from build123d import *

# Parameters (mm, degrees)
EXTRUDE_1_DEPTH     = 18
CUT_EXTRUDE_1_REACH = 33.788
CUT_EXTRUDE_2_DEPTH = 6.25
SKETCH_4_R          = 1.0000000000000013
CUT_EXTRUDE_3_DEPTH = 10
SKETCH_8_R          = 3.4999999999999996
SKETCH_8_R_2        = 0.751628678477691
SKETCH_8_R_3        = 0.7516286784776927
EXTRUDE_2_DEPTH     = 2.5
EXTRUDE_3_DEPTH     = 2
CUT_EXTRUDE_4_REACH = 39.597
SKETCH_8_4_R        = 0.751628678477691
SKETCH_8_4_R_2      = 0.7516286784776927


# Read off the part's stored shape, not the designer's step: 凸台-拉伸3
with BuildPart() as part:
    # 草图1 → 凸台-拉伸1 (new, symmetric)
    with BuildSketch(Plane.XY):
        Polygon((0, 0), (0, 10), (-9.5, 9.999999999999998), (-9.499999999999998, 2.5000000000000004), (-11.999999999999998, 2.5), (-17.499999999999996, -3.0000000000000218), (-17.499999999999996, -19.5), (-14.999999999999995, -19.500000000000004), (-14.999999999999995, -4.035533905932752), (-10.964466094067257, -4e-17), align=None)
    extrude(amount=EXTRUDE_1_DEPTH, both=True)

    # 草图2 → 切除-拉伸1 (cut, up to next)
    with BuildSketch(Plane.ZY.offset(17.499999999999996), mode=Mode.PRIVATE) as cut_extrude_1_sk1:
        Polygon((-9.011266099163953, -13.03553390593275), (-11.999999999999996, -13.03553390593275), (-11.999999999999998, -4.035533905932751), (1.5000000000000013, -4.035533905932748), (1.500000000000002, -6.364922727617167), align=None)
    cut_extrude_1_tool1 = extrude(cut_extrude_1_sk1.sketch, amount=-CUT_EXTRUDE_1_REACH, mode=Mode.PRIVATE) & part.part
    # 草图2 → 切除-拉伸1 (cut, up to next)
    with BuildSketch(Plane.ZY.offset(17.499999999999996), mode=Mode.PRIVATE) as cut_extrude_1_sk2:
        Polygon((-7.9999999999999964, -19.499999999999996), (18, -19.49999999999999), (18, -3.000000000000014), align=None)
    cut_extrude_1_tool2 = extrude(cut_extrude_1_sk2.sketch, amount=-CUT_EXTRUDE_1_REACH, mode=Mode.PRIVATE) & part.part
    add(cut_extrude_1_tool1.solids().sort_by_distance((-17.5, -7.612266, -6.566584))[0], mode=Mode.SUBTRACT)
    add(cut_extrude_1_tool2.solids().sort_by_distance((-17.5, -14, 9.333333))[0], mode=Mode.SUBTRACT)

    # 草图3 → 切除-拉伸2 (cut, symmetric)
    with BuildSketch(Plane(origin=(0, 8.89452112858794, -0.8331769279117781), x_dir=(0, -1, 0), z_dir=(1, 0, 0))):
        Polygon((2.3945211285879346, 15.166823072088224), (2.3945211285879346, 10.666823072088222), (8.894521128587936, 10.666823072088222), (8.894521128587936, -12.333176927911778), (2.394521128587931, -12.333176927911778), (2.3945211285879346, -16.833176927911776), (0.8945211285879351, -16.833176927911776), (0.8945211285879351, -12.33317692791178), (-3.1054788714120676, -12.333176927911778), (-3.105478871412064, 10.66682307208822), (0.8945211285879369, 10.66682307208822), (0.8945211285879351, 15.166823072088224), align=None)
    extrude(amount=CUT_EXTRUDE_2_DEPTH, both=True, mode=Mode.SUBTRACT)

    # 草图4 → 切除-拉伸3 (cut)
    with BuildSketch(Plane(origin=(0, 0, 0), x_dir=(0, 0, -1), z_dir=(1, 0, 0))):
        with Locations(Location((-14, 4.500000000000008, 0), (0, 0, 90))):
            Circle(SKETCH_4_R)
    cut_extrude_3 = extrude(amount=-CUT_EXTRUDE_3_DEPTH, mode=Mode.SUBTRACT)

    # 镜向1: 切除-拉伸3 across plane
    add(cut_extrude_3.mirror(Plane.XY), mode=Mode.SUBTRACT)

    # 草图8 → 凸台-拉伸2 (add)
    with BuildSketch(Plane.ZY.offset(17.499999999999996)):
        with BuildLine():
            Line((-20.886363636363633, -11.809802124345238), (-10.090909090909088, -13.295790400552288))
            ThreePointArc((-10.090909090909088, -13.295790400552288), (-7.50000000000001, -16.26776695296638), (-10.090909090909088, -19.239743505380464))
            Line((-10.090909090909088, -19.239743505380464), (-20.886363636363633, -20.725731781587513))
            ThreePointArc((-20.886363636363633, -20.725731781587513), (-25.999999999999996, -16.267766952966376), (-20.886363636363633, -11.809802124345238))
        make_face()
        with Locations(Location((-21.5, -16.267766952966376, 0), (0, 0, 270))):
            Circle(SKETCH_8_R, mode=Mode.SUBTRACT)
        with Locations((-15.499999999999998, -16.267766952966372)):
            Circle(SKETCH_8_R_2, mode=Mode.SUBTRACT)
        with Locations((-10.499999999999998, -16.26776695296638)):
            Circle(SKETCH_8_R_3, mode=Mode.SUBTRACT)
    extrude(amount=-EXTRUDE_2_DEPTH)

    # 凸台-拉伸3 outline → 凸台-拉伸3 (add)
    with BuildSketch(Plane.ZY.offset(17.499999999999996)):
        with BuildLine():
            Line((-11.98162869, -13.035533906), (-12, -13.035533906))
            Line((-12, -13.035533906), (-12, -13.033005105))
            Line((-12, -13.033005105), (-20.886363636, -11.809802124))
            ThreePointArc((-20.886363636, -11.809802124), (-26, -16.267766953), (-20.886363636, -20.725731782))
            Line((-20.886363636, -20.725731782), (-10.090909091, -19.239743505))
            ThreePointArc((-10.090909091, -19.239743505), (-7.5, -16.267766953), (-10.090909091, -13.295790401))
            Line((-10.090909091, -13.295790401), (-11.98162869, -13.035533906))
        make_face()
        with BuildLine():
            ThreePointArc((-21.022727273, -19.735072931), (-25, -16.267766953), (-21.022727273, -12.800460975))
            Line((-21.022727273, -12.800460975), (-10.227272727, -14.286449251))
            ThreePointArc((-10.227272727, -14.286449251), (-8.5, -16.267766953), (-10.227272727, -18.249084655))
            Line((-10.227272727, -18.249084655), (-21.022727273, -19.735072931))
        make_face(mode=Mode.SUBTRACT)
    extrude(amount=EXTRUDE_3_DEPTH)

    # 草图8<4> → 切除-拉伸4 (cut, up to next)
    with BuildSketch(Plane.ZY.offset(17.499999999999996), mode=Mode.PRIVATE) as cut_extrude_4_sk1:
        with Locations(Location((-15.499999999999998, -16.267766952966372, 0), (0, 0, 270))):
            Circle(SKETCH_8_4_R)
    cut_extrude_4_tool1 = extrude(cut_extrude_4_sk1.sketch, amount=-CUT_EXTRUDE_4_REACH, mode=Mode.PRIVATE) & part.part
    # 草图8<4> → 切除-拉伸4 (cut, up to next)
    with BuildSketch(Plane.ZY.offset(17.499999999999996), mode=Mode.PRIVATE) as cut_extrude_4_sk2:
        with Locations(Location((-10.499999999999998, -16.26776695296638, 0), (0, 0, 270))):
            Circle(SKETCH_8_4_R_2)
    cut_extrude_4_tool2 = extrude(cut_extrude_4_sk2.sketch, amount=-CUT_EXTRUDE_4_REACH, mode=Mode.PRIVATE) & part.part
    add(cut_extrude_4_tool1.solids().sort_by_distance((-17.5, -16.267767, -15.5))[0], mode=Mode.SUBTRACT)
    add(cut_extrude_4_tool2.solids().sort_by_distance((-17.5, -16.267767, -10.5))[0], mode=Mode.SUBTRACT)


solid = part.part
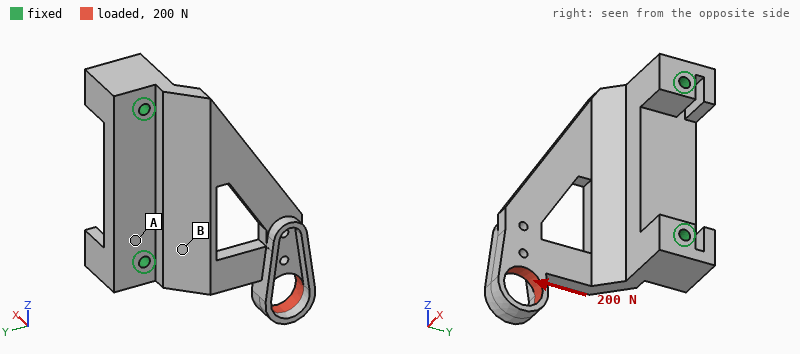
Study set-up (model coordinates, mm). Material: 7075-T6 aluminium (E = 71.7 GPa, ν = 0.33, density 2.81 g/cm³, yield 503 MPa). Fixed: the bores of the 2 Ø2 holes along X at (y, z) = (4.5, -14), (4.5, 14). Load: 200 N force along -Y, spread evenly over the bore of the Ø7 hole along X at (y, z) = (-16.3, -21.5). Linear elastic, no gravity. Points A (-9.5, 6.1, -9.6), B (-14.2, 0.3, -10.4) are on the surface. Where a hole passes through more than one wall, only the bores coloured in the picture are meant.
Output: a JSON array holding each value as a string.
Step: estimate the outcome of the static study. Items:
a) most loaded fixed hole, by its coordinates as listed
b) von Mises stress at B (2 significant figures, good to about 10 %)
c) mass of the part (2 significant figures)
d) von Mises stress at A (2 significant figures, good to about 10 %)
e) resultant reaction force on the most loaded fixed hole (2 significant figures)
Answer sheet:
["(4.5, -14)", "52 MPa", "9.7 g", "13 MPa", "250 N"]
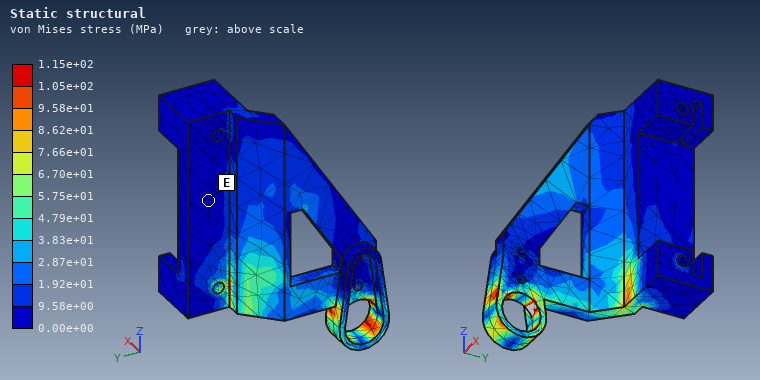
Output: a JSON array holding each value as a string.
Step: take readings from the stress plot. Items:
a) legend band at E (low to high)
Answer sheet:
["0.00e+00 to 9.58e+00 MPa"]
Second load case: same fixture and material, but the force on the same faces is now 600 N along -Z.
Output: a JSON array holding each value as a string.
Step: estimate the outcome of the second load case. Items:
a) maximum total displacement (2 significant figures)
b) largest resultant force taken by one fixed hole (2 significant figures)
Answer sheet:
["0.20 mm", "560 N"]
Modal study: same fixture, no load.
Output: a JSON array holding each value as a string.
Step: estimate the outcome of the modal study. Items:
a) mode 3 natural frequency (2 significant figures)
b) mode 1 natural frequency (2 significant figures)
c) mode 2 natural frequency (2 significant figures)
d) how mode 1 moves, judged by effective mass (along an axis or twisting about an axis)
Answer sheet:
["10 kHz", "3000 Hz", "7600 Hz", "along X"]
